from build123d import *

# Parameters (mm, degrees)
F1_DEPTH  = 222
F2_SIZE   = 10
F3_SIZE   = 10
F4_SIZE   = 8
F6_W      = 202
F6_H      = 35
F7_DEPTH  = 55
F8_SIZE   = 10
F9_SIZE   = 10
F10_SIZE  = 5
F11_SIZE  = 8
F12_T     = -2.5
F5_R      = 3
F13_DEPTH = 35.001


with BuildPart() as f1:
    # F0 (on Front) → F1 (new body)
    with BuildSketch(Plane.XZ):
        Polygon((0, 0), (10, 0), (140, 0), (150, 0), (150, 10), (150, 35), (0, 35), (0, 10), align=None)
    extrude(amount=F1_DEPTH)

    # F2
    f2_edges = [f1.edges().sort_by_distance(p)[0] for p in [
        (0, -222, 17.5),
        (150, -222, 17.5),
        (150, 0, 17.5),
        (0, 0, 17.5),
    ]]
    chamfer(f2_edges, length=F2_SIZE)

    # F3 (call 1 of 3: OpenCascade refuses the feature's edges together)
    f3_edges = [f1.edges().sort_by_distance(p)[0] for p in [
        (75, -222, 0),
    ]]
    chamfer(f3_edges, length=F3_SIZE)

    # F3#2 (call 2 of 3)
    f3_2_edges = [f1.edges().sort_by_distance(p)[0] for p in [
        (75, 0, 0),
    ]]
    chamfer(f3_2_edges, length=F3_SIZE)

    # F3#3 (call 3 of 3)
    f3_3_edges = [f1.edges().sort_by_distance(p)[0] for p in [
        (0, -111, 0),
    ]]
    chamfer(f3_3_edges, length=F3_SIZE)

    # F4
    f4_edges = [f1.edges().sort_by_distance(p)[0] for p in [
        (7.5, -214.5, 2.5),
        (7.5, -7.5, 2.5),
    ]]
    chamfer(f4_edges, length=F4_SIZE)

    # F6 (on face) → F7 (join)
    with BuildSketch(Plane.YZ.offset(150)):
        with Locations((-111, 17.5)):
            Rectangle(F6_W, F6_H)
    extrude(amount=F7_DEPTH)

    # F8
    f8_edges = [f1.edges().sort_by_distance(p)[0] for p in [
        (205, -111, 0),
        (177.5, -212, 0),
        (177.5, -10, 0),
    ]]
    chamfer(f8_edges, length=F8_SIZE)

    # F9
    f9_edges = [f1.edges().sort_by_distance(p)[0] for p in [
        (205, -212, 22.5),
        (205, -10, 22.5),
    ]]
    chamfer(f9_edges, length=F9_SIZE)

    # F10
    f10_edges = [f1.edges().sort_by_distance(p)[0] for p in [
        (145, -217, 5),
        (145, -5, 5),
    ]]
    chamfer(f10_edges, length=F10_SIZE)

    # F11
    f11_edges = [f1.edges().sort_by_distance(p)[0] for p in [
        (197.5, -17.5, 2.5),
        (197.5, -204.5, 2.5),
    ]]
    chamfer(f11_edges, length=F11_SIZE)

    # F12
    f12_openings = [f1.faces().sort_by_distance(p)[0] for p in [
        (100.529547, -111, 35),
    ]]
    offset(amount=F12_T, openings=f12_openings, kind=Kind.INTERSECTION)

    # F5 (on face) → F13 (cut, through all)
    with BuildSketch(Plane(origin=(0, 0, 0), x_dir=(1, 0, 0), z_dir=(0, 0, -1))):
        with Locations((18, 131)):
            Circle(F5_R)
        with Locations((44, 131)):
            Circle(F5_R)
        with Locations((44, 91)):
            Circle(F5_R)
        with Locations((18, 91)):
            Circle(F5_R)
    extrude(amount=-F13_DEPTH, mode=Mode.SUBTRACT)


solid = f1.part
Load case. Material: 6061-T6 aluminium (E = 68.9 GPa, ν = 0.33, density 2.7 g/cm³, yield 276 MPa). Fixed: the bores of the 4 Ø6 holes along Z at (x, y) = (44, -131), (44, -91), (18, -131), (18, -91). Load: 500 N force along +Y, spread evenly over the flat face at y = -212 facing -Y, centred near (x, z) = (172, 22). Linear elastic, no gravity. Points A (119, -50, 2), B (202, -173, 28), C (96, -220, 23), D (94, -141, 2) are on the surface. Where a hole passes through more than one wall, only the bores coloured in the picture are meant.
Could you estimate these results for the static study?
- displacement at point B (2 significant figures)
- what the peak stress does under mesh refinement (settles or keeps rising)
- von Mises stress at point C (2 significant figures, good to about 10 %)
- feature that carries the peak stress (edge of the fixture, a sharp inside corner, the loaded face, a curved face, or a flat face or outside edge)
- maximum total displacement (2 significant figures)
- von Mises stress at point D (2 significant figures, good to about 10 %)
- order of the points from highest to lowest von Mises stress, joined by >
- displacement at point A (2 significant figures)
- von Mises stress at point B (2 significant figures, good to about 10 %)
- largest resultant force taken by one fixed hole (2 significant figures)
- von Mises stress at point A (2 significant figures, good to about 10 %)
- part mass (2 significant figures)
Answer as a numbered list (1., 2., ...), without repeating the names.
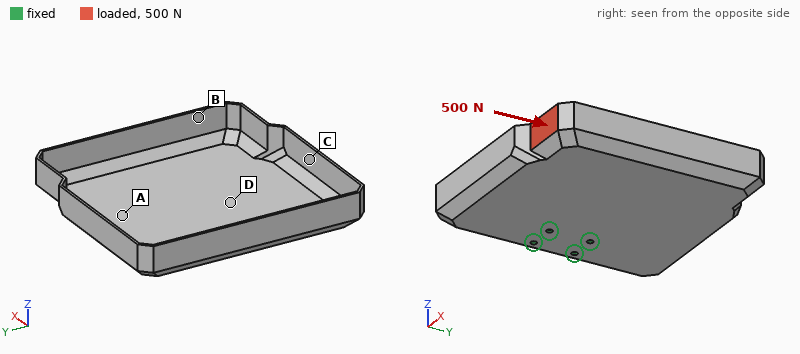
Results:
1. 2.0 mm
2. keeps rising
3. 27 MPa
4. edge of the fixture
5. 3.0 mm
6. 21 MPa
7. C > D > A > B
8. 0.77 mm
9. 11 MPa
10. 970 N
11. 14 MPa
12. 440 g
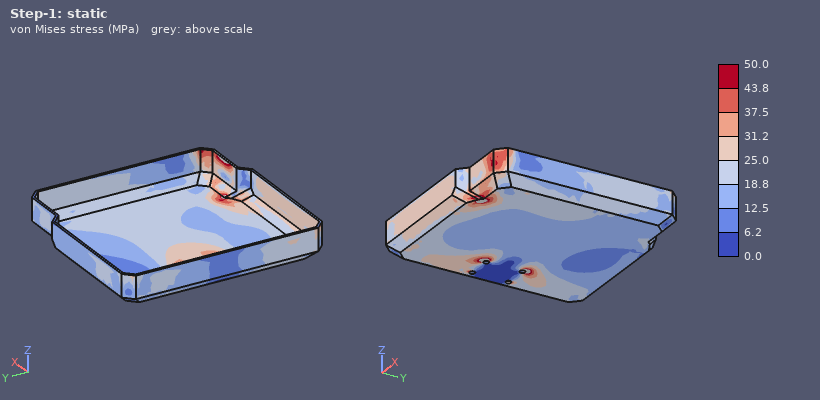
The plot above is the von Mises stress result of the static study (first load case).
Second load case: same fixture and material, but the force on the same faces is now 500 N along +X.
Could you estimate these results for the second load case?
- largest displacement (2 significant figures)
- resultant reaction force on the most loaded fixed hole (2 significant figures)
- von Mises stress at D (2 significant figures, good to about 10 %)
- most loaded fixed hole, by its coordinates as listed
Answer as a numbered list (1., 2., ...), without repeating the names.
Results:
1. 3.4 mm
2. 820 N
3. 15 MPa
4. (44, -131)
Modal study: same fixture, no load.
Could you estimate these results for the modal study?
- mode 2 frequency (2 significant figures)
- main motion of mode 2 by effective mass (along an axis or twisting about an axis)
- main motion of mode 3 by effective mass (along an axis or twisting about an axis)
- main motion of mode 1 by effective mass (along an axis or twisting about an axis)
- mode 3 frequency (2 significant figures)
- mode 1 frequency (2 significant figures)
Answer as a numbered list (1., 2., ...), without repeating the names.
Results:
1. 110 Hz
2. twisting about X
3. twisting about X
4. along Z
5. 530 Hz
6. 77 Hz
